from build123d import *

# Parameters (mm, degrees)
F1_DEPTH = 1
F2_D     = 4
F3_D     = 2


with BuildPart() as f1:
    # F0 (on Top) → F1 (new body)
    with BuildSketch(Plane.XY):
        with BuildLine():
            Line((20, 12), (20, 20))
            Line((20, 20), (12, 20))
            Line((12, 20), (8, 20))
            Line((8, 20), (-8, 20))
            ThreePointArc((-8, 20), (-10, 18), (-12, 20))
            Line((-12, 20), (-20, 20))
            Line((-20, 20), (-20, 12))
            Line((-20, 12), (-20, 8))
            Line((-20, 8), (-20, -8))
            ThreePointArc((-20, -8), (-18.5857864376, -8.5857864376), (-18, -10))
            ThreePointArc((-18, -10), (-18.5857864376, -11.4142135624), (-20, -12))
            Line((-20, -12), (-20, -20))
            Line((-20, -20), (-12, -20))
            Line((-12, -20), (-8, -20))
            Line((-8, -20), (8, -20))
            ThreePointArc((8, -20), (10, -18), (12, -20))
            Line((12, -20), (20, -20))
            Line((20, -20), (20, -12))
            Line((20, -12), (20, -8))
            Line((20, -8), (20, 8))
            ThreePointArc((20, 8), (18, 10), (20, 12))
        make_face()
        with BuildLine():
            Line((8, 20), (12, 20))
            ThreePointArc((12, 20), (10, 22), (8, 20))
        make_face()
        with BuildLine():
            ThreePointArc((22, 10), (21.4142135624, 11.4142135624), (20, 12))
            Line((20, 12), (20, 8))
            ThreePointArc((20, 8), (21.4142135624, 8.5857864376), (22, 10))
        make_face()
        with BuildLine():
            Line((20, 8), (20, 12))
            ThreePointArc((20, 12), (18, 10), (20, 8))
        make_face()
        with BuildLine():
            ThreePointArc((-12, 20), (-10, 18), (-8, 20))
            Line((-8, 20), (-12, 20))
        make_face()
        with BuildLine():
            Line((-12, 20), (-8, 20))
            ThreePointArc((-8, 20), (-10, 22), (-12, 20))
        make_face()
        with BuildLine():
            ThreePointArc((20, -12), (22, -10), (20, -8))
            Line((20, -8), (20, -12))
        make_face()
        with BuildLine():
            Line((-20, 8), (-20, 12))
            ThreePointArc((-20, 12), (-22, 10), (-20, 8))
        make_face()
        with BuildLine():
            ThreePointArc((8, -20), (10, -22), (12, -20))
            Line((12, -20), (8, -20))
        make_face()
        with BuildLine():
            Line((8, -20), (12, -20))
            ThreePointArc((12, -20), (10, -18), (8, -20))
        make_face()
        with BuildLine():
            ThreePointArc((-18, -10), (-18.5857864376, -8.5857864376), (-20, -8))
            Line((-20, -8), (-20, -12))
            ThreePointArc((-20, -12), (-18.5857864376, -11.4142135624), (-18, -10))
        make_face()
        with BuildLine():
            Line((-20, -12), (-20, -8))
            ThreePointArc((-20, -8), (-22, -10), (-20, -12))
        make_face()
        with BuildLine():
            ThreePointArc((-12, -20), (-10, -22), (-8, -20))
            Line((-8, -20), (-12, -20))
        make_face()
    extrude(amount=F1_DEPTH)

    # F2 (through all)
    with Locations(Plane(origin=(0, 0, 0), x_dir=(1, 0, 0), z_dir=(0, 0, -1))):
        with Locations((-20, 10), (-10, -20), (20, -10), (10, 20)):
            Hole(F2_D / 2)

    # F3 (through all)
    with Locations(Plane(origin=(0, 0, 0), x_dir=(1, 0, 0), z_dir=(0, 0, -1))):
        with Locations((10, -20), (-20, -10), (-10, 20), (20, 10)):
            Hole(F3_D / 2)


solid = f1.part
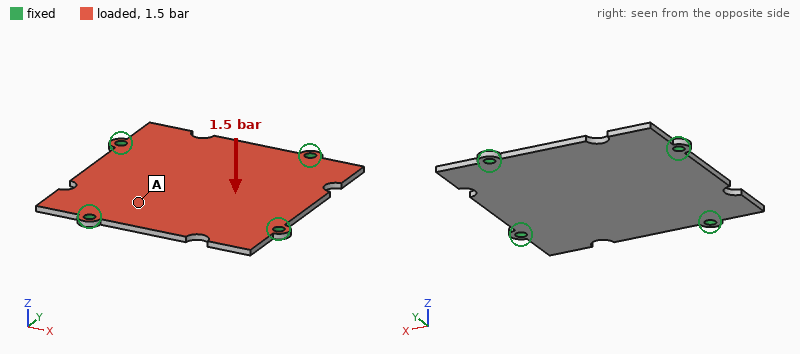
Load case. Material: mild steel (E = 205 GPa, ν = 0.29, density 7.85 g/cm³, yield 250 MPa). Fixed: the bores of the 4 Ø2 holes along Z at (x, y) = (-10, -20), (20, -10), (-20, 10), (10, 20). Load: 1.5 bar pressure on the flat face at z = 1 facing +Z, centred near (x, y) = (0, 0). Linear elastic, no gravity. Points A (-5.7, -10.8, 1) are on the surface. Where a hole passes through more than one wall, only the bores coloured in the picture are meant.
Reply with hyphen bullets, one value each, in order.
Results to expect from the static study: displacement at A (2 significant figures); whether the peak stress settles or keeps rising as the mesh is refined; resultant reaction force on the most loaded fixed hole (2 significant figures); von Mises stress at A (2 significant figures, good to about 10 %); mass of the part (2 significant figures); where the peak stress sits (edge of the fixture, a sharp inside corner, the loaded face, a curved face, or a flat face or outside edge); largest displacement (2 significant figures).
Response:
- 36 µm
- keeps rising
- 60 N
- 26 MPa
- 12 g
- edge of the fixture
- 60 µm
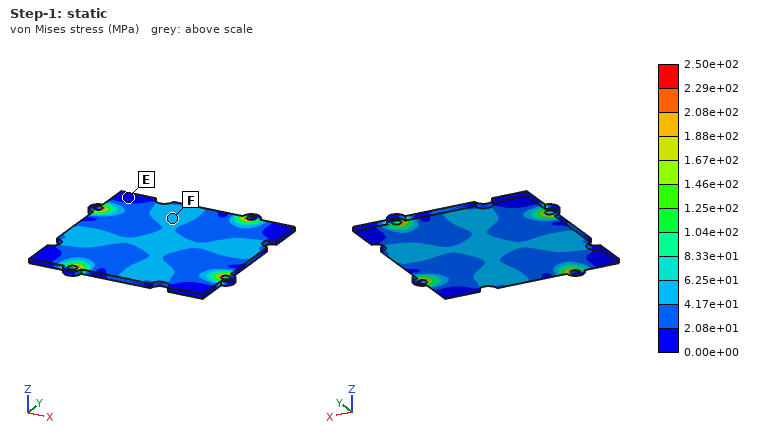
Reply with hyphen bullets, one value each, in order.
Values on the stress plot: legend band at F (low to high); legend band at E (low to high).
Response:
- 4.17e+01 to 6.25e+01 MPa
- 0.00e+00 to 2.08e+01 MPa
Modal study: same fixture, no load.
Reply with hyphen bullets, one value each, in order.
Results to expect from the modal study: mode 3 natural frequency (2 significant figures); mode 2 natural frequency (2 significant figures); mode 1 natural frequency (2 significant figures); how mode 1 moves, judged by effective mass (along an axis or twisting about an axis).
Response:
- 5200 Hz
- 5000 Hz
- 3400 Hz
- along Z
